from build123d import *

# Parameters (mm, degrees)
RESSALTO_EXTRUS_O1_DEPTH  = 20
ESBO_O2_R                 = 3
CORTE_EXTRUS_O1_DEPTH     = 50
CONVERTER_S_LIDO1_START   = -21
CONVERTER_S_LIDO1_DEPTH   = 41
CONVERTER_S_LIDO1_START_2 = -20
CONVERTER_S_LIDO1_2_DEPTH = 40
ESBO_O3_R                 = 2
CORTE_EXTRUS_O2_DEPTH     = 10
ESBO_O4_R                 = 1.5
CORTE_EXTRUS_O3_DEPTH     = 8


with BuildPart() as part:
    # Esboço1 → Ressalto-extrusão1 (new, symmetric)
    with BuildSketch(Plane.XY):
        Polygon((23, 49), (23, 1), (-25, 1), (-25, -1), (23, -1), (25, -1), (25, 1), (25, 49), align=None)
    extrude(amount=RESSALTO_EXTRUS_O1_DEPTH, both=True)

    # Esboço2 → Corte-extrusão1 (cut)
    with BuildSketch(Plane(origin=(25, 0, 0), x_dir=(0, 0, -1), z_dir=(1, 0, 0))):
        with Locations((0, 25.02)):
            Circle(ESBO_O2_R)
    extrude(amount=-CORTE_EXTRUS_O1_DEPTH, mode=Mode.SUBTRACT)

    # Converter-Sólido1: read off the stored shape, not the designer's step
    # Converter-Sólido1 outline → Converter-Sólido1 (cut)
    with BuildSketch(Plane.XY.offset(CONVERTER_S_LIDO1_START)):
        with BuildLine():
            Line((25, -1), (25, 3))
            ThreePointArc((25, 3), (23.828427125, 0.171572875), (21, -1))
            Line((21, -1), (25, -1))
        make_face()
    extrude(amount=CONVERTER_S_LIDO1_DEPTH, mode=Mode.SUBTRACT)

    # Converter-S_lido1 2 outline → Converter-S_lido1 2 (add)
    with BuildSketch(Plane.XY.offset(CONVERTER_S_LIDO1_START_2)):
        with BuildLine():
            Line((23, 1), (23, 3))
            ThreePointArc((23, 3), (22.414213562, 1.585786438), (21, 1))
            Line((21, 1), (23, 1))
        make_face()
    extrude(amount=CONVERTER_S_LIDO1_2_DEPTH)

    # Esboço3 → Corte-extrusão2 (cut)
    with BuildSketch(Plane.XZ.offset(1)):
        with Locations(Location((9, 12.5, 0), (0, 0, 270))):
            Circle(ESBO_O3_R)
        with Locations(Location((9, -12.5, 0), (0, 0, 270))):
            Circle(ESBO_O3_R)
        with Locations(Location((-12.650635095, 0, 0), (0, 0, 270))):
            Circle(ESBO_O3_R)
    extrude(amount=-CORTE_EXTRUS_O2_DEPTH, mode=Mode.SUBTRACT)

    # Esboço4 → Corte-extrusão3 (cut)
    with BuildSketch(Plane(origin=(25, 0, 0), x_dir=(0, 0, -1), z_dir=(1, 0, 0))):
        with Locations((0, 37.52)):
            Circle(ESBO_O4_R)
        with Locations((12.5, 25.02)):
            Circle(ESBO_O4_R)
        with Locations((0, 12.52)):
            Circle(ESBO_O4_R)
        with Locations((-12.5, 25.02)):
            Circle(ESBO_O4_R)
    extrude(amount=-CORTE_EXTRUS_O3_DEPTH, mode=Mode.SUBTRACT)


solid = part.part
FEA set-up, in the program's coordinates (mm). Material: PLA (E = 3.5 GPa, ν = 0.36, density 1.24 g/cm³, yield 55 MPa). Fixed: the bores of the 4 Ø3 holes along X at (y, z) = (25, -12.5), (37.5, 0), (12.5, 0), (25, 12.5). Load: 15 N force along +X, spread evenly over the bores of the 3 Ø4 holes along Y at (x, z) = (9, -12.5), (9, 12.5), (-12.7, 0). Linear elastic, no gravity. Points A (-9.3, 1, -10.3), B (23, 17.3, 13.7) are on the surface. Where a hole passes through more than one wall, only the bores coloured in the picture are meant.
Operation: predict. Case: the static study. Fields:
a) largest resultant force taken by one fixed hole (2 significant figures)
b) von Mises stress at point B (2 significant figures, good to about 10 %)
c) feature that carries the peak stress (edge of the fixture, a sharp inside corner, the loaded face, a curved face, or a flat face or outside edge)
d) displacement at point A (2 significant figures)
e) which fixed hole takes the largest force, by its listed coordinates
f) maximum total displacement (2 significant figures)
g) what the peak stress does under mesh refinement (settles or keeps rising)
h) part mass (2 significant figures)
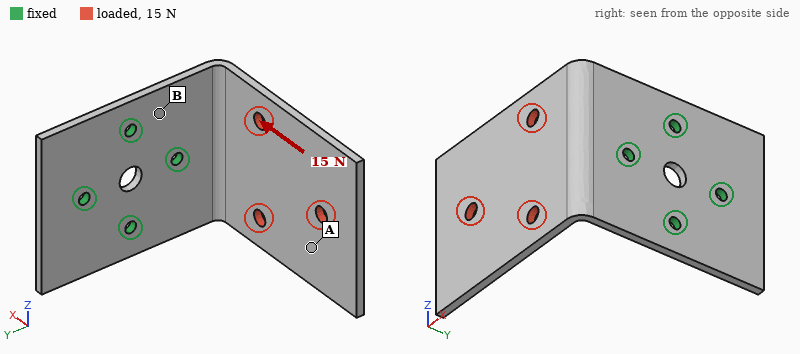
20 N
2.0 MPa
edge of the fixture
0.51 mm
(12.5, 0)
0.75 mm
keeps rising
9.4 g
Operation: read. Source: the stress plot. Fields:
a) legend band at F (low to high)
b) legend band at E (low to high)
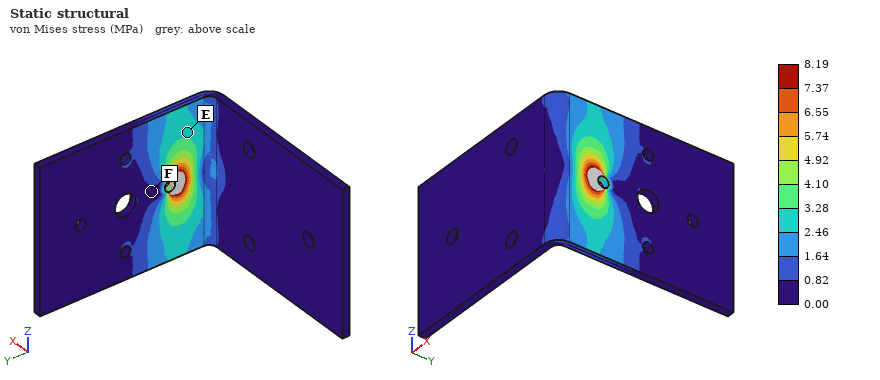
0.00 to 0.82 MPa
2.46 to 3.28 MPa
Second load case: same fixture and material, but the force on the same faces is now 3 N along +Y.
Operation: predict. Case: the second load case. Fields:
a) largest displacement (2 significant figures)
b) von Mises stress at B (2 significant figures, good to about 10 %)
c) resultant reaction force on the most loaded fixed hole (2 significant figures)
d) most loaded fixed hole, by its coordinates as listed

0.76 mm
0.73 MPa
3.4 N
(12.5, 0)
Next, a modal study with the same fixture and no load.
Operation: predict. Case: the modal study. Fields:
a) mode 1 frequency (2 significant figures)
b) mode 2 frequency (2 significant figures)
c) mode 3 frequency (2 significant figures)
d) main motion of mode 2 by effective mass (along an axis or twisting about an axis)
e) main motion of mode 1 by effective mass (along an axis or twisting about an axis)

160 Hz
280 Hz
600 Hz
along Z
along Y
